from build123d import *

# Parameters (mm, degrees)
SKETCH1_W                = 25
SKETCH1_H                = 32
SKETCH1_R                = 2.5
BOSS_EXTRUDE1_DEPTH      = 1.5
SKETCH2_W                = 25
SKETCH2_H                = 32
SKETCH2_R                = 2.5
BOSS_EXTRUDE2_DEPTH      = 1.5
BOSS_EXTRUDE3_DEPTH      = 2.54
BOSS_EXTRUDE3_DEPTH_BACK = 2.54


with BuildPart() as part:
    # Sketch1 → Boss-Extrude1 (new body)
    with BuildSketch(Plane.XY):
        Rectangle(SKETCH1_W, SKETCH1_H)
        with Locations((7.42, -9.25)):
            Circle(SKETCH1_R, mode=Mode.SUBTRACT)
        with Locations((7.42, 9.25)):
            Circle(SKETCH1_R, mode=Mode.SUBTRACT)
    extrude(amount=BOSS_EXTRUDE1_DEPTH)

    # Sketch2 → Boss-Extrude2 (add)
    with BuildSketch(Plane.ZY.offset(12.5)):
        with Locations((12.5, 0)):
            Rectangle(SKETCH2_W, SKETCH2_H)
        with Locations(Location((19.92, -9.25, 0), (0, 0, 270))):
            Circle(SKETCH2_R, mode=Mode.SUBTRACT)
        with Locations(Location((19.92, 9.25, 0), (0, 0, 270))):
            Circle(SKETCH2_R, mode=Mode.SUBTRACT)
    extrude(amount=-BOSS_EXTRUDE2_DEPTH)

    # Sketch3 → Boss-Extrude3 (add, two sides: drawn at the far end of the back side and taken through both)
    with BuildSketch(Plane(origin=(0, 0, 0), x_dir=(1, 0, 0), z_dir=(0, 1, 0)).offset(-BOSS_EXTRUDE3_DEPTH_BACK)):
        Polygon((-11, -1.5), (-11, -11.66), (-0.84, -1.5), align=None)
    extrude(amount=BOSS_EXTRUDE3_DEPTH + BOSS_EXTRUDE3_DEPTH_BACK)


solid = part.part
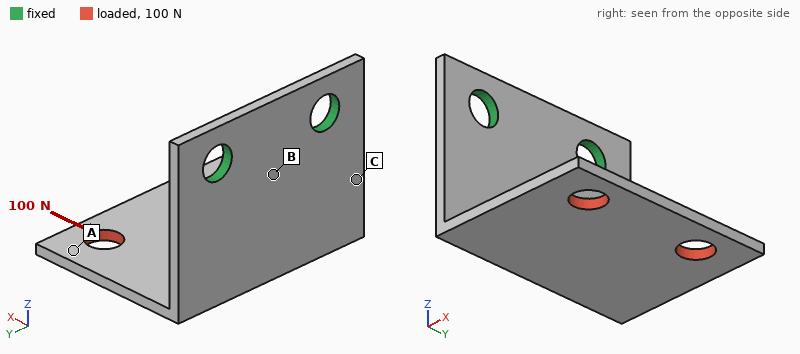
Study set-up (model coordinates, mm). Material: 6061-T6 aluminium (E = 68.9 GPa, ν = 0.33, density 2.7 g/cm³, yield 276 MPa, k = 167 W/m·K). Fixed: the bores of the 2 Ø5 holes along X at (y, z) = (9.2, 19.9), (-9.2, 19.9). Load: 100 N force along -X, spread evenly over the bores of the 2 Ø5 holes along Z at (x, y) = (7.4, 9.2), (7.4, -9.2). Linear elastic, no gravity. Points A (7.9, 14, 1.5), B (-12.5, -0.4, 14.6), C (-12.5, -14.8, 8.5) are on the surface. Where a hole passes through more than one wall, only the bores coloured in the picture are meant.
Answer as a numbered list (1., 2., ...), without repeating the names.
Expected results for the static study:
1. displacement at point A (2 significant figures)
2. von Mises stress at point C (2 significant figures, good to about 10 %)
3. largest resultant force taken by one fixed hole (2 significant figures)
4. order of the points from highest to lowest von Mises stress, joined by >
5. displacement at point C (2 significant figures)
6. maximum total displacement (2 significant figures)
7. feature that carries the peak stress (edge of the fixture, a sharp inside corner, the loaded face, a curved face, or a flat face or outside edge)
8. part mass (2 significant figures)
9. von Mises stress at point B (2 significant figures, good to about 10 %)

1. 0.44 mm
2. 51 MPa
3. 50 N
4. B > C > A
5. 0.10 mm
6. 0.52 mm
7. a flat face or outside edge
8. 6.7 g
9. 88 MPa
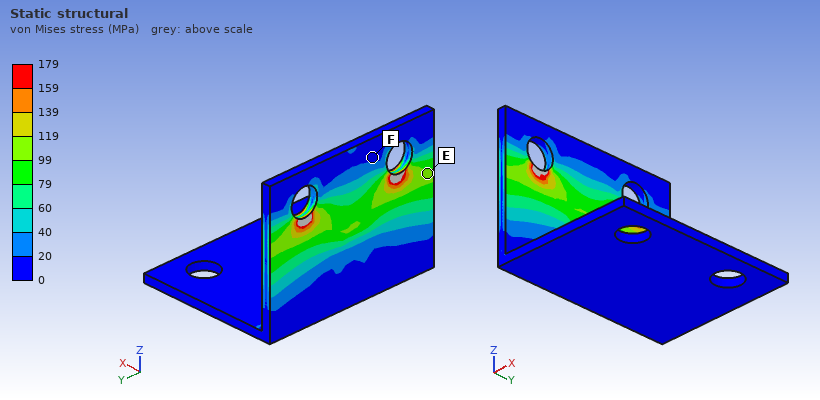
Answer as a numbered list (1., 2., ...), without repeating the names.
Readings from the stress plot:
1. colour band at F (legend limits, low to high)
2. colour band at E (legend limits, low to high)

1. 0 to 20 MPa
2. 99 to 119 MPa
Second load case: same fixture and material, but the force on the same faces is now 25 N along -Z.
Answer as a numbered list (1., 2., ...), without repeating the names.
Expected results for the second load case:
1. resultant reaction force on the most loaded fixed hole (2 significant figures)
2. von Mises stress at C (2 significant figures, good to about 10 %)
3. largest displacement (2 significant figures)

1. 14 N
2. 21 MPa
3. 0.23 mm
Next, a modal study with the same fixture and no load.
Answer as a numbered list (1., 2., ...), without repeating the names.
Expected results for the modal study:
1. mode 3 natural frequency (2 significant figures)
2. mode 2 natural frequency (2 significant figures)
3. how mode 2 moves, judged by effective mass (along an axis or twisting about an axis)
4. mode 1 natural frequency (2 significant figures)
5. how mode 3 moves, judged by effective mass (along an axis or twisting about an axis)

1. 4500 Hz
2. 2300 Hz
3. along Y
4. 1200 Hz
5. along X
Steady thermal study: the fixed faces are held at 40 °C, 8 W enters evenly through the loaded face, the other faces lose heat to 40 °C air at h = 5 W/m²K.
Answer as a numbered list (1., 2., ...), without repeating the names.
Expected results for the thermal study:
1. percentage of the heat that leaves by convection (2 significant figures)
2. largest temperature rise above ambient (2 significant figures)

1. 3.2 %
2. 35 K
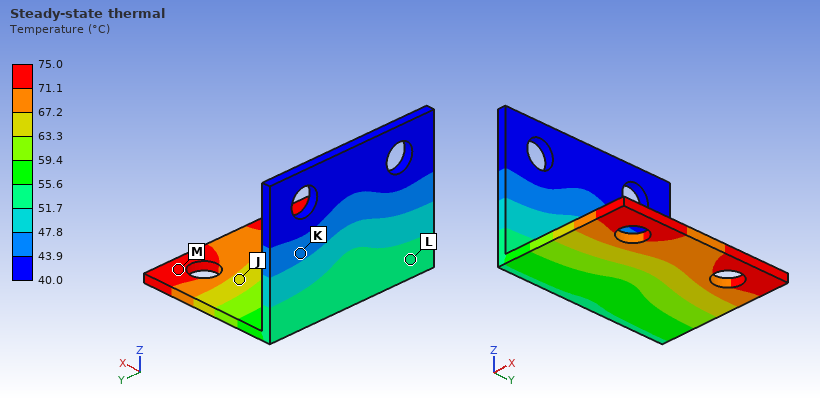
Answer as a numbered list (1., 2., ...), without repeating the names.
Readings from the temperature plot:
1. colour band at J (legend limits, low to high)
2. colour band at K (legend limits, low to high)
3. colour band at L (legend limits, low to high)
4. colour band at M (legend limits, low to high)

1. 63.3 to 67.2 °C
2. 43.9 to 47.8 °C
3. 51.7 to 55.6 °C
4. 71.1 to 75.0 °C
